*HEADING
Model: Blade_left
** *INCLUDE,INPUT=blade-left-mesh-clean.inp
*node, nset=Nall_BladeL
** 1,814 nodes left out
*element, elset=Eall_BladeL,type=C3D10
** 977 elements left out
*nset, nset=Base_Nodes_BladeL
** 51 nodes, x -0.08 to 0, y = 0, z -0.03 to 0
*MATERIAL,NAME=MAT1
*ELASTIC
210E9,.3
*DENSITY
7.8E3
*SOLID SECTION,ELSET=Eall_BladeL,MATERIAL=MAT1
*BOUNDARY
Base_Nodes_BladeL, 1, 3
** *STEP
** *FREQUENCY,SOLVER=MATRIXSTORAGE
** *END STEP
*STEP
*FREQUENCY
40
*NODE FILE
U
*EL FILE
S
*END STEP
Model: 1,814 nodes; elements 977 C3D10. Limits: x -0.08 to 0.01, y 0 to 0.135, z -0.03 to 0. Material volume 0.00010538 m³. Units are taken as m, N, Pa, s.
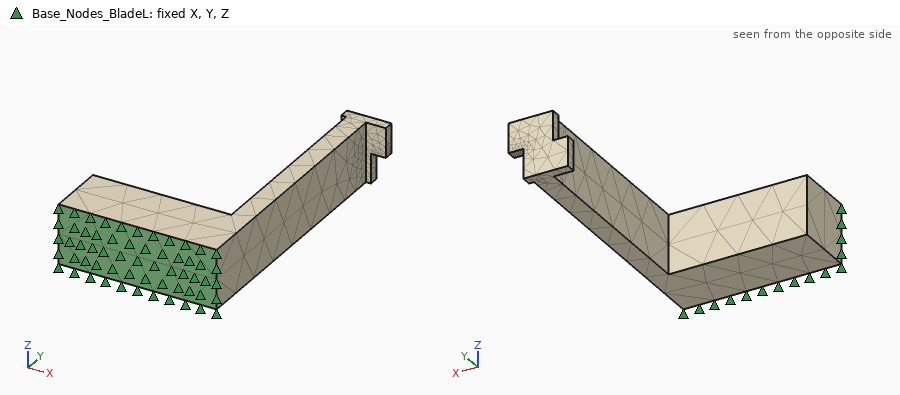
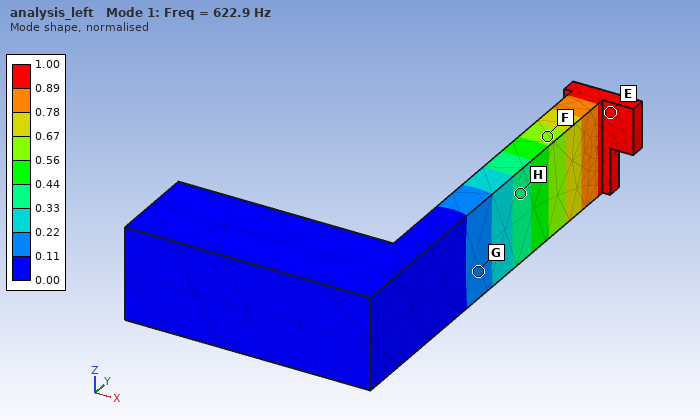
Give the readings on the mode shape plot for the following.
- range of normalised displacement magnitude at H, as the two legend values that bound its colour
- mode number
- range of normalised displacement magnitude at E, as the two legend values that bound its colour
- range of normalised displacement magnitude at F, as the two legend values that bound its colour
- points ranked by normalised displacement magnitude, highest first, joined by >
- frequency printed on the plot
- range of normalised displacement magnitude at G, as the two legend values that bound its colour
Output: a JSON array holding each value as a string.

["0.33 to 0.44", "1", "0.89 to 1.00", "0.56 to 0.67", "E > F > H > G", "622.9 Hz", "0.11 to 0.22"]
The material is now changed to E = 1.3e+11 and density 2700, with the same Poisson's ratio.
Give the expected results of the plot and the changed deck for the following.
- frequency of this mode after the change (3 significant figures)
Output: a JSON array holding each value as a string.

["833 Hz"]
